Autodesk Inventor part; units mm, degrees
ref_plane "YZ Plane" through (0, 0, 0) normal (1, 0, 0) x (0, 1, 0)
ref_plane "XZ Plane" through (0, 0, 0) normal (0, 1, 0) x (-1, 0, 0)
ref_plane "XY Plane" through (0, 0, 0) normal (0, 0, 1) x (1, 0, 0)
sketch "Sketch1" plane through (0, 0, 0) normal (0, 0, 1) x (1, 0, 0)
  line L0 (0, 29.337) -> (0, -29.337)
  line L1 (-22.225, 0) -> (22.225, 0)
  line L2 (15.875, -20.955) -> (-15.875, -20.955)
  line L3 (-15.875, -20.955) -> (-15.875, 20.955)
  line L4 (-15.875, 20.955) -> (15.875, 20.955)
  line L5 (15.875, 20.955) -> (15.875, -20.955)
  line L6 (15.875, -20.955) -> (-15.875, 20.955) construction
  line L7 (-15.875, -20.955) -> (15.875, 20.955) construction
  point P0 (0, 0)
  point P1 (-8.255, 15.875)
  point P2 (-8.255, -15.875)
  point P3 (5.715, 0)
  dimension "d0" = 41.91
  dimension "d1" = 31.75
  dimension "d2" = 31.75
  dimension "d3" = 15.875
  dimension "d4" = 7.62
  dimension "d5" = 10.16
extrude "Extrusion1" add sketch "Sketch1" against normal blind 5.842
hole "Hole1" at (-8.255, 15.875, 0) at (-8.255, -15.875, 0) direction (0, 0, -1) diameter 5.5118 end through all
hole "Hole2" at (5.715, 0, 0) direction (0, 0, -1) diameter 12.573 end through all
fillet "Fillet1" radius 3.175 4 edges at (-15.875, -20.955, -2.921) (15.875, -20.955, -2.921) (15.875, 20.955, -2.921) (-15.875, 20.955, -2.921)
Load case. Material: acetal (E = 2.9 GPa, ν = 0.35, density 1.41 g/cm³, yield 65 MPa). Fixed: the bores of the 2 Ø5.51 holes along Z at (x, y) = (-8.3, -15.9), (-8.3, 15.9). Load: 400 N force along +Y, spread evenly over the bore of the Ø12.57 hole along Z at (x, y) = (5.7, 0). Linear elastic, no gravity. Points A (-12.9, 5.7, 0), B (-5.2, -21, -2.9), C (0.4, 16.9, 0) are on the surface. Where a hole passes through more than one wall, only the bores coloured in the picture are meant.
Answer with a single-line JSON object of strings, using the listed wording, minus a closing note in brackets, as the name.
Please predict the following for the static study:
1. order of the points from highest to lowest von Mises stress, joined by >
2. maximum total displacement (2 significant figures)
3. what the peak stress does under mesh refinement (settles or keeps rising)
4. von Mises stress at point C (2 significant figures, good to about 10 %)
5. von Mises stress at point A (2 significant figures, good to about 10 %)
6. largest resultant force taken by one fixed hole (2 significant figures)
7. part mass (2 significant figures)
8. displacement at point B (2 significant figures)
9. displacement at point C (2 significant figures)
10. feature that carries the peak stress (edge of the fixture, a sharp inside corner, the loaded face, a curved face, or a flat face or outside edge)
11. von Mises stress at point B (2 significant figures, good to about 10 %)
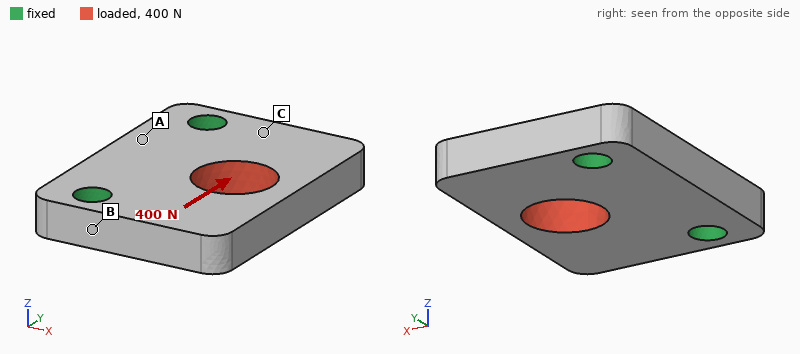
{"order of the points from highest to lowest von Mises stress, joined by >": "B > C > A", "maximum total displacement": "60 µm", "what the peak stress does under mesh refinement": "keeps rising", "von Mises stress at point C": "2.6 MPa", "von Mises stress at point A": "0.89 MPa", "largest resultant force taken by one fixed hole": "250 N", "part mass": "9.5 g", "displacement at point B": "9.3 µm", "displacement at point C": "19 µm", "feature that carries the peak stress": "edge of the fixture", "von Mises stress at point B": "4.6 MPa"}
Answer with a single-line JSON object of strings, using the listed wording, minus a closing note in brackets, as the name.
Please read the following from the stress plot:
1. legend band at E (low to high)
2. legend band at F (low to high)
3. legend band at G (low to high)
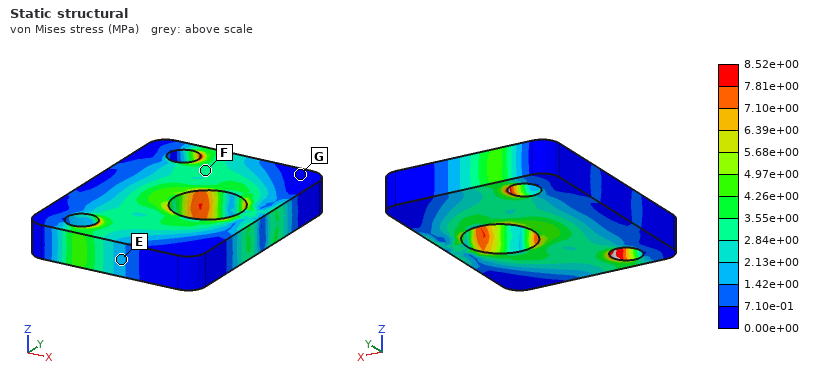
{"legend band at E": "1.42e+00 to 2.13e+00 MPa", "legend band at F": "2.84e+00 to 3.55e+00 MPa", "legend band at G": "0.00e+00 to 7.10e-01 MPa"}
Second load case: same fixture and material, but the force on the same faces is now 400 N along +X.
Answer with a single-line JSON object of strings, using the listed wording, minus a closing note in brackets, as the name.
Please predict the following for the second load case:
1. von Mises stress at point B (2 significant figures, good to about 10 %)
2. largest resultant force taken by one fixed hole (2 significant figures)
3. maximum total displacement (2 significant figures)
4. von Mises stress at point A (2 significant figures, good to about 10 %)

{"von Mises stress at point B": "0.88 MPa", "largest resultant force taken by one fixed hole": "210 N", "maximum total displacement": "37 µm", "von Mises stress at point A": "1.1 MPa"}
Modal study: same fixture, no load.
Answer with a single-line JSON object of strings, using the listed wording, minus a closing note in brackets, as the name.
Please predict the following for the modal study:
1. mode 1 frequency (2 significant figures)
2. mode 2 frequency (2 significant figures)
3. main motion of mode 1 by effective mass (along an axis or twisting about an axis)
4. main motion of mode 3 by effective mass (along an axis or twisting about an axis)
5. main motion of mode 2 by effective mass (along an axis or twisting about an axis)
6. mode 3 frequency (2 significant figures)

{"mode 1 frequency": "2200 Hz", "mode 2 frequency": "3600 Hz", "main motion of mode 1 by effective mass": "along Z", "main motion of mode 3 by effective mass": "along Y", "main motion of mode 2 by effective mass": "twisting about X", "mode 3 frequency": "6200 Hz"}
